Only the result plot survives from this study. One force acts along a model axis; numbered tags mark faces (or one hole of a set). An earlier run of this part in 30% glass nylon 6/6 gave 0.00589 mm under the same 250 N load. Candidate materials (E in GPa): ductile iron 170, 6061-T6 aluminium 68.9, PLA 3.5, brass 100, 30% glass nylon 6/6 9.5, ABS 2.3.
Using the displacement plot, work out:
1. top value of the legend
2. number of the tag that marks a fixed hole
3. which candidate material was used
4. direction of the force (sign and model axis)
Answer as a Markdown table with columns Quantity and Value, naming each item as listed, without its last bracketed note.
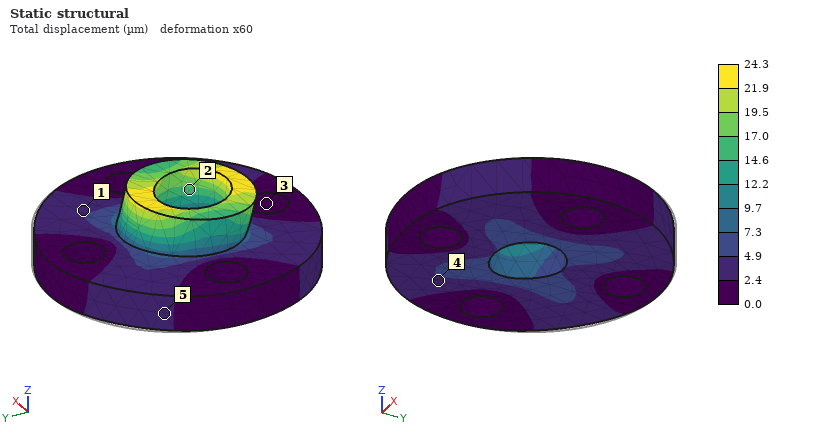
| Quantity | Value |
|---|---|
| top value of the legend | 24.3 µm |
| number of the tag that marks a fixed hole | 3 |
| which candidate material was used | ABS |
| direction of the force | -Y |
